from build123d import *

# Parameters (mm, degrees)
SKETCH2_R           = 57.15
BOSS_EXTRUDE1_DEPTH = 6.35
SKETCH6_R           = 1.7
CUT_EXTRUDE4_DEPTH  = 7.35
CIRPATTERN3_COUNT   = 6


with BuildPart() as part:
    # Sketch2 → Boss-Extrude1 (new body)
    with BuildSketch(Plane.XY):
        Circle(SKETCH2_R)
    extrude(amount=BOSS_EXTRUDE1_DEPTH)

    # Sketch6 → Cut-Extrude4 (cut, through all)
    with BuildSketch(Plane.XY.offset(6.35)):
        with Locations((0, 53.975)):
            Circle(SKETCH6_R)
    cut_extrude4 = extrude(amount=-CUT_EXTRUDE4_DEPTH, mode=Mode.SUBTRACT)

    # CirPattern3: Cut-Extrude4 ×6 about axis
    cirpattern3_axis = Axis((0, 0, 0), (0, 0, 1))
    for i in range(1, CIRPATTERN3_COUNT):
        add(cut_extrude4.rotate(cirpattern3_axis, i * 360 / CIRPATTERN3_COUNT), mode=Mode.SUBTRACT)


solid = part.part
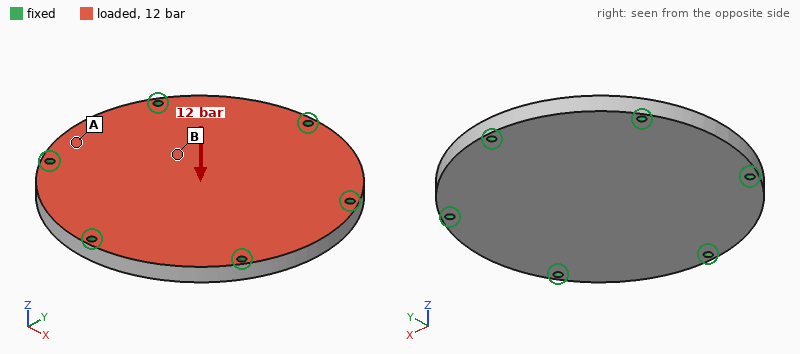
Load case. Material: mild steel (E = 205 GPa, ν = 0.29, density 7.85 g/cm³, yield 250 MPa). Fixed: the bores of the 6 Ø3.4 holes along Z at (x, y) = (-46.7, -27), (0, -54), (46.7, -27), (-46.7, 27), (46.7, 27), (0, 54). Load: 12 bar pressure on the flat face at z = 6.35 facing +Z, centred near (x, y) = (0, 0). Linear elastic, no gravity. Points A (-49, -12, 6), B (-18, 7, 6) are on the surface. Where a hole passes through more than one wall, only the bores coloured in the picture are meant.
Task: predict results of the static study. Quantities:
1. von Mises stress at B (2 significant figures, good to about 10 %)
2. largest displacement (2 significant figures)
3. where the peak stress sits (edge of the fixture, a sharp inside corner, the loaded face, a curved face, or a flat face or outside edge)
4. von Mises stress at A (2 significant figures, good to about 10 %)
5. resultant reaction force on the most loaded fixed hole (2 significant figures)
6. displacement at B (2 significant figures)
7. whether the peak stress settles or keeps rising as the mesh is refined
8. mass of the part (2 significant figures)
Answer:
45 MPa
62 µm
edge of the fixture
26 MPa
2.0 kN
51 µm
keeps rising
510 g
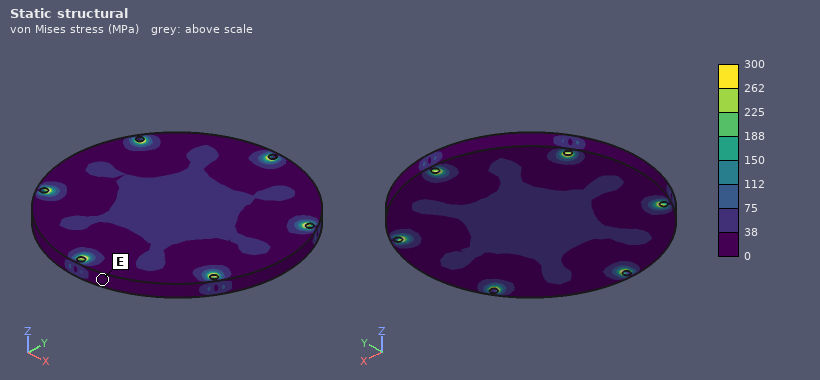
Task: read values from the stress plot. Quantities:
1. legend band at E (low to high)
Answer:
0 to 38 MPa
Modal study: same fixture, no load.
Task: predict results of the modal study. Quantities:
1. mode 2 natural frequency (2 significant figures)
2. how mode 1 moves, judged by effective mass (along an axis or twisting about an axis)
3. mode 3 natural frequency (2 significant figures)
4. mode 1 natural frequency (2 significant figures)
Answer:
7900 Hz
along Z
7900 Hz
3900 Hz
